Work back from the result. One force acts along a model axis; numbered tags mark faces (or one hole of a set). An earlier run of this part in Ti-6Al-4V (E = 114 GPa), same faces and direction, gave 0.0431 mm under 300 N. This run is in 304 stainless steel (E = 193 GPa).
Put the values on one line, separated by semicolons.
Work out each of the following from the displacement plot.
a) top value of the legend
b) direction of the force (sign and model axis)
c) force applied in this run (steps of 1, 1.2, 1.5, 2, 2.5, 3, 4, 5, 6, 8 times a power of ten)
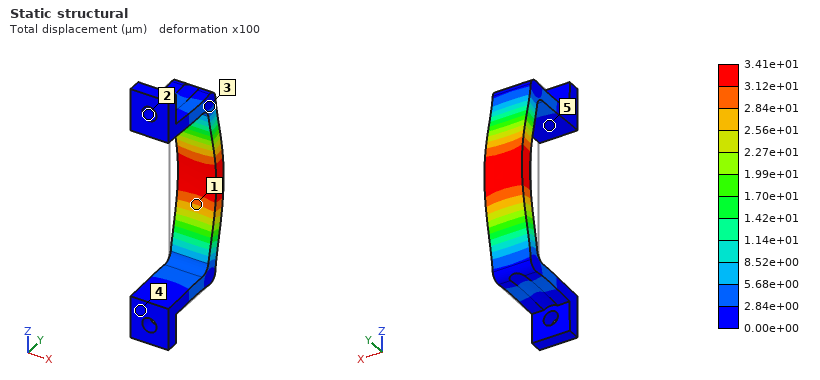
3.41e+01 µm; +Y; 400 N
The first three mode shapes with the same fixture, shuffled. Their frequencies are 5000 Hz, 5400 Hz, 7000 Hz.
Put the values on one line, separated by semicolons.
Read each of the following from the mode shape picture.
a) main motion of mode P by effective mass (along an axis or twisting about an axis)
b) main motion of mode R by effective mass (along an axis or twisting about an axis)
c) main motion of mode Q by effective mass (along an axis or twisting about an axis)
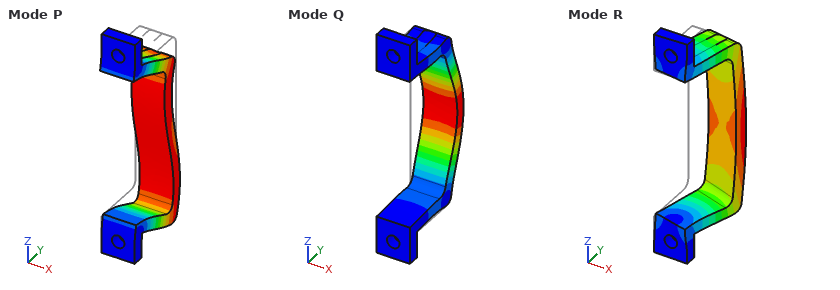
along Z; along X; along Y
